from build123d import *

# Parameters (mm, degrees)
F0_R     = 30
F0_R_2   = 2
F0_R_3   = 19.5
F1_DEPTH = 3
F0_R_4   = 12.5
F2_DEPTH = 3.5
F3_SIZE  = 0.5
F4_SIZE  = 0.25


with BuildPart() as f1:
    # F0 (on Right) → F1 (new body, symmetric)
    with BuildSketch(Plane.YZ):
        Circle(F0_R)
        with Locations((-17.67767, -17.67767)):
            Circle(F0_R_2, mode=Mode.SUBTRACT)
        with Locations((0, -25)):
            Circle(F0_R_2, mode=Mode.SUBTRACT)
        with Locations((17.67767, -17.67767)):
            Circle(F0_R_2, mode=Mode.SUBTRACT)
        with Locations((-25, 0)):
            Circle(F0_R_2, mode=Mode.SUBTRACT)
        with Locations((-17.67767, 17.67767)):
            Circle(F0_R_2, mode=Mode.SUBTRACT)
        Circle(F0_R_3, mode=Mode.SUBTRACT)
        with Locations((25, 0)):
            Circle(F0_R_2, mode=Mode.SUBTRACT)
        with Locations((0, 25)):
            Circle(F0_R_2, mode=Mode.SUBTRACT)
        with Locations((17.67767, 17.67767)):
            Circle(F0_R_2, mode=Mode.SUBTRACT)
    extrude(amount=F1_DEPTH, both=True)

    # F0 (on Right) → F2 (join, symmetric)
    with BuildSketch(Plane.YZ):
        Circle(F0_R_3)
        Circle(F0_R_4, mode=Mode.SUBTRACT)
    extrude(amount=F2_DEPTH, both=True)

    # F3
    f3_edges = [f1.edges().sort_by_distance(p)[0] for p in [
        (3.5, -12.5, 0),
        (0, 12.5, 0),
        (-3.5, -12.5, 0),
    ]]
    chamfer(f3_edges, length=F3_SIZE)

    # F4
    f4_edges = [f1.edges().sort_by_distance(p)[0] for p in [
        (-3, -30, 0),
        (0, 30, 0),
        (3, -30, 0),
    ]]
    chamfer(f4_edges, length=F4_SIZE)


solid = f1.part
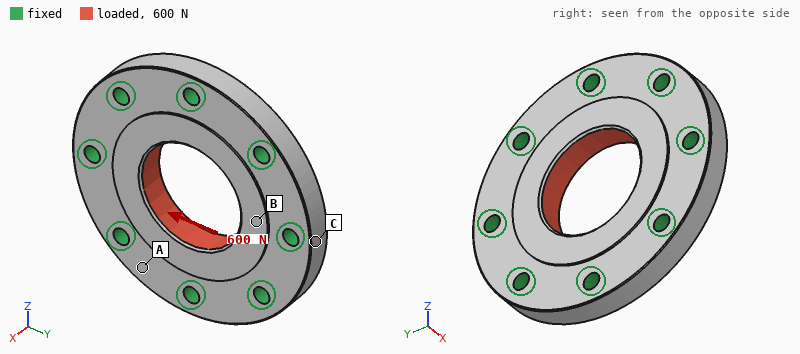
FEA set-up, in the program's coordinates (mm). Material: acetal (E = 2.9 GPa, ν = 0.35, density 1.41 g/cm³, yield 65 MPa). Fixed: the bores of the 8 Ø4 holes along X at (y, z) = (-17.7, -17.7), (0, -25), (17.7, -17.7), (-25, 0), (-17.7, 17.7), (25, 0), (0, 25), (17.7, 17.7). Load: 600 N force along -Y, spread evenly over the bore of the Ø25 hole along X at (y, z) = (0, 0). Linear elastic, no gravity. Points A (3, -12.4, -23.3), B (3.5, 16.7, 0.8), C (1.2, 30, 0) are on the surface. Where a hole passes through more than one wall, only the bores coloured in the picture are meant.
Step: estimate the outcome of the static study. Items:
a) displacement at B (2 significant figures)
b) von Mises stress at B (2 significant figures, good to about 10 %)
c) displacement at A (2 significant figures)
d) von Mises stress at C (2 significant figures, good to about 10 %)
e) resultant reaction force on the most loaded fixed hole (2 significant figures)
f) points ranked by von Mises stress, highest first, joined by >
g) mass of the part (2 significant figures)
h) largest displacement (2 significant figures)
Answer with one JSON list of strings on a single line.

["4.3 µm", "1.2 MPa", "1.4 µm", "0.71 MPa", "110 N", "B > C > A", "20 g", "7.0 µm"]
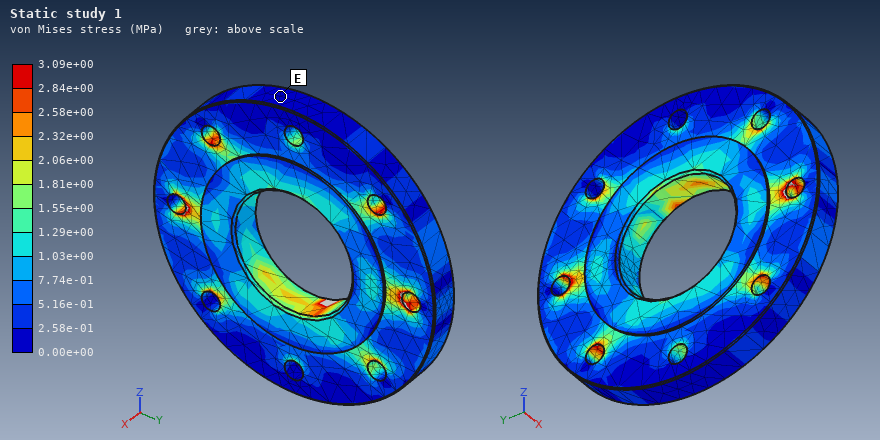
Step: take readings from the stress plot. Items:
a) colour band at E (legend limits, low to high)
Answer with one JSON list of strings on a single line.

["0.00e+00 to 2.58e-01 MPa"]
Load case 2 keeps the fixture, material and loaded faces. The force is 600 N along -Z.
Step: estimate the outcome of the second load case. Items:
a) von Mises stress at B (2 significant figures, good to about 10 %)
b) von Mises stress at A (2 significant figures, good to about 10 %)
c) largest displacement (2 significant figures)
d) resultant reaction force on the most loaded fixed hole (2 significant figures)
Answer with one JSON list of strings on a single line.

["0.76 MPa", "0.45 MPa", "6.9 µm", "110 N"]
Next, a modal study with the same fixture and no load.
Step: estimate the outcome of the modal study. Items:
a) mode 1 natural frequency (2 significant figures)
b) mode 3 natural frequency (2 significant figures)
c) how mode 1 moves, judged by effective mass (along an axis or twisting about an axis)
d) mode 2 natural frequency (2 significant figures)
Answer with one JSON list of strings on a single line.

["8400 Hz", "10 kHz", "along X", "10 kHz"]
